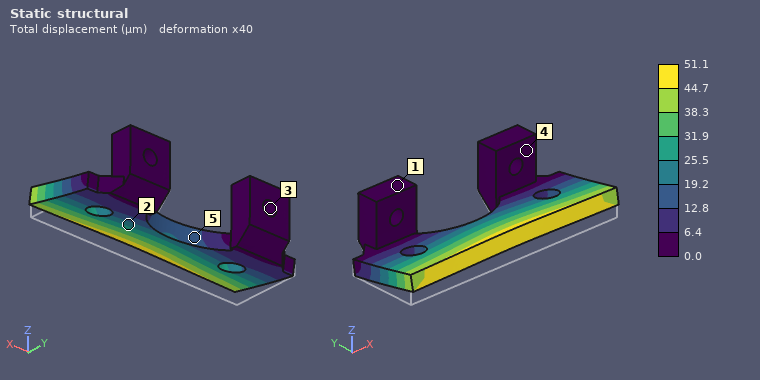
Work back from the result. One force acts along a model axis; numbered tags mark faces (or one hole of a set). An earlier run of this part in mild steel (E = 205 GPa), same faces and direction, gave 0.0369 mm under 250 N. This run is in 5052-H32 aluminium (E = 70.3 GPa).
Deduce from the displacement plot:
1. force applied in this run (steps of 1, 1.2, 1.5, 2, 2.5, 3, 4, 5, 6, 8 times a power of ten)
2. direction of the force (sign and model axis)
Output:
120 N
+Z
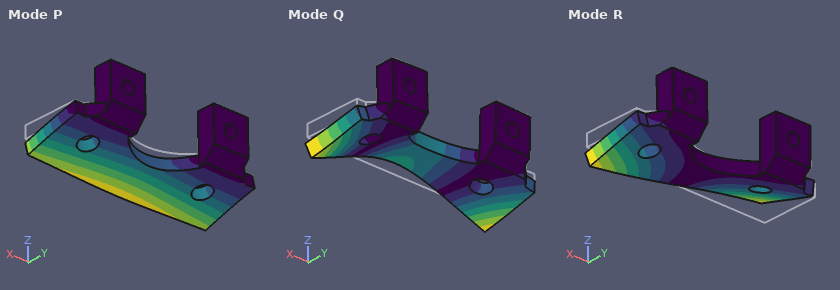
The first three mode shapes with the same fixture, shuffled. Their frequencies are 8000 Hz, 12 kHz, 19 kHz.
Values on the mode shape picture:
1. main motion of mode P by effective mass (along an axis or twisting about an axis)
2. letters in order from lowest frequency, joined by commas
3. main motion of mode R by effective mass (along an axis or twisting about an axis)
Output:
along Z
P, R, Q
twisting about Y
